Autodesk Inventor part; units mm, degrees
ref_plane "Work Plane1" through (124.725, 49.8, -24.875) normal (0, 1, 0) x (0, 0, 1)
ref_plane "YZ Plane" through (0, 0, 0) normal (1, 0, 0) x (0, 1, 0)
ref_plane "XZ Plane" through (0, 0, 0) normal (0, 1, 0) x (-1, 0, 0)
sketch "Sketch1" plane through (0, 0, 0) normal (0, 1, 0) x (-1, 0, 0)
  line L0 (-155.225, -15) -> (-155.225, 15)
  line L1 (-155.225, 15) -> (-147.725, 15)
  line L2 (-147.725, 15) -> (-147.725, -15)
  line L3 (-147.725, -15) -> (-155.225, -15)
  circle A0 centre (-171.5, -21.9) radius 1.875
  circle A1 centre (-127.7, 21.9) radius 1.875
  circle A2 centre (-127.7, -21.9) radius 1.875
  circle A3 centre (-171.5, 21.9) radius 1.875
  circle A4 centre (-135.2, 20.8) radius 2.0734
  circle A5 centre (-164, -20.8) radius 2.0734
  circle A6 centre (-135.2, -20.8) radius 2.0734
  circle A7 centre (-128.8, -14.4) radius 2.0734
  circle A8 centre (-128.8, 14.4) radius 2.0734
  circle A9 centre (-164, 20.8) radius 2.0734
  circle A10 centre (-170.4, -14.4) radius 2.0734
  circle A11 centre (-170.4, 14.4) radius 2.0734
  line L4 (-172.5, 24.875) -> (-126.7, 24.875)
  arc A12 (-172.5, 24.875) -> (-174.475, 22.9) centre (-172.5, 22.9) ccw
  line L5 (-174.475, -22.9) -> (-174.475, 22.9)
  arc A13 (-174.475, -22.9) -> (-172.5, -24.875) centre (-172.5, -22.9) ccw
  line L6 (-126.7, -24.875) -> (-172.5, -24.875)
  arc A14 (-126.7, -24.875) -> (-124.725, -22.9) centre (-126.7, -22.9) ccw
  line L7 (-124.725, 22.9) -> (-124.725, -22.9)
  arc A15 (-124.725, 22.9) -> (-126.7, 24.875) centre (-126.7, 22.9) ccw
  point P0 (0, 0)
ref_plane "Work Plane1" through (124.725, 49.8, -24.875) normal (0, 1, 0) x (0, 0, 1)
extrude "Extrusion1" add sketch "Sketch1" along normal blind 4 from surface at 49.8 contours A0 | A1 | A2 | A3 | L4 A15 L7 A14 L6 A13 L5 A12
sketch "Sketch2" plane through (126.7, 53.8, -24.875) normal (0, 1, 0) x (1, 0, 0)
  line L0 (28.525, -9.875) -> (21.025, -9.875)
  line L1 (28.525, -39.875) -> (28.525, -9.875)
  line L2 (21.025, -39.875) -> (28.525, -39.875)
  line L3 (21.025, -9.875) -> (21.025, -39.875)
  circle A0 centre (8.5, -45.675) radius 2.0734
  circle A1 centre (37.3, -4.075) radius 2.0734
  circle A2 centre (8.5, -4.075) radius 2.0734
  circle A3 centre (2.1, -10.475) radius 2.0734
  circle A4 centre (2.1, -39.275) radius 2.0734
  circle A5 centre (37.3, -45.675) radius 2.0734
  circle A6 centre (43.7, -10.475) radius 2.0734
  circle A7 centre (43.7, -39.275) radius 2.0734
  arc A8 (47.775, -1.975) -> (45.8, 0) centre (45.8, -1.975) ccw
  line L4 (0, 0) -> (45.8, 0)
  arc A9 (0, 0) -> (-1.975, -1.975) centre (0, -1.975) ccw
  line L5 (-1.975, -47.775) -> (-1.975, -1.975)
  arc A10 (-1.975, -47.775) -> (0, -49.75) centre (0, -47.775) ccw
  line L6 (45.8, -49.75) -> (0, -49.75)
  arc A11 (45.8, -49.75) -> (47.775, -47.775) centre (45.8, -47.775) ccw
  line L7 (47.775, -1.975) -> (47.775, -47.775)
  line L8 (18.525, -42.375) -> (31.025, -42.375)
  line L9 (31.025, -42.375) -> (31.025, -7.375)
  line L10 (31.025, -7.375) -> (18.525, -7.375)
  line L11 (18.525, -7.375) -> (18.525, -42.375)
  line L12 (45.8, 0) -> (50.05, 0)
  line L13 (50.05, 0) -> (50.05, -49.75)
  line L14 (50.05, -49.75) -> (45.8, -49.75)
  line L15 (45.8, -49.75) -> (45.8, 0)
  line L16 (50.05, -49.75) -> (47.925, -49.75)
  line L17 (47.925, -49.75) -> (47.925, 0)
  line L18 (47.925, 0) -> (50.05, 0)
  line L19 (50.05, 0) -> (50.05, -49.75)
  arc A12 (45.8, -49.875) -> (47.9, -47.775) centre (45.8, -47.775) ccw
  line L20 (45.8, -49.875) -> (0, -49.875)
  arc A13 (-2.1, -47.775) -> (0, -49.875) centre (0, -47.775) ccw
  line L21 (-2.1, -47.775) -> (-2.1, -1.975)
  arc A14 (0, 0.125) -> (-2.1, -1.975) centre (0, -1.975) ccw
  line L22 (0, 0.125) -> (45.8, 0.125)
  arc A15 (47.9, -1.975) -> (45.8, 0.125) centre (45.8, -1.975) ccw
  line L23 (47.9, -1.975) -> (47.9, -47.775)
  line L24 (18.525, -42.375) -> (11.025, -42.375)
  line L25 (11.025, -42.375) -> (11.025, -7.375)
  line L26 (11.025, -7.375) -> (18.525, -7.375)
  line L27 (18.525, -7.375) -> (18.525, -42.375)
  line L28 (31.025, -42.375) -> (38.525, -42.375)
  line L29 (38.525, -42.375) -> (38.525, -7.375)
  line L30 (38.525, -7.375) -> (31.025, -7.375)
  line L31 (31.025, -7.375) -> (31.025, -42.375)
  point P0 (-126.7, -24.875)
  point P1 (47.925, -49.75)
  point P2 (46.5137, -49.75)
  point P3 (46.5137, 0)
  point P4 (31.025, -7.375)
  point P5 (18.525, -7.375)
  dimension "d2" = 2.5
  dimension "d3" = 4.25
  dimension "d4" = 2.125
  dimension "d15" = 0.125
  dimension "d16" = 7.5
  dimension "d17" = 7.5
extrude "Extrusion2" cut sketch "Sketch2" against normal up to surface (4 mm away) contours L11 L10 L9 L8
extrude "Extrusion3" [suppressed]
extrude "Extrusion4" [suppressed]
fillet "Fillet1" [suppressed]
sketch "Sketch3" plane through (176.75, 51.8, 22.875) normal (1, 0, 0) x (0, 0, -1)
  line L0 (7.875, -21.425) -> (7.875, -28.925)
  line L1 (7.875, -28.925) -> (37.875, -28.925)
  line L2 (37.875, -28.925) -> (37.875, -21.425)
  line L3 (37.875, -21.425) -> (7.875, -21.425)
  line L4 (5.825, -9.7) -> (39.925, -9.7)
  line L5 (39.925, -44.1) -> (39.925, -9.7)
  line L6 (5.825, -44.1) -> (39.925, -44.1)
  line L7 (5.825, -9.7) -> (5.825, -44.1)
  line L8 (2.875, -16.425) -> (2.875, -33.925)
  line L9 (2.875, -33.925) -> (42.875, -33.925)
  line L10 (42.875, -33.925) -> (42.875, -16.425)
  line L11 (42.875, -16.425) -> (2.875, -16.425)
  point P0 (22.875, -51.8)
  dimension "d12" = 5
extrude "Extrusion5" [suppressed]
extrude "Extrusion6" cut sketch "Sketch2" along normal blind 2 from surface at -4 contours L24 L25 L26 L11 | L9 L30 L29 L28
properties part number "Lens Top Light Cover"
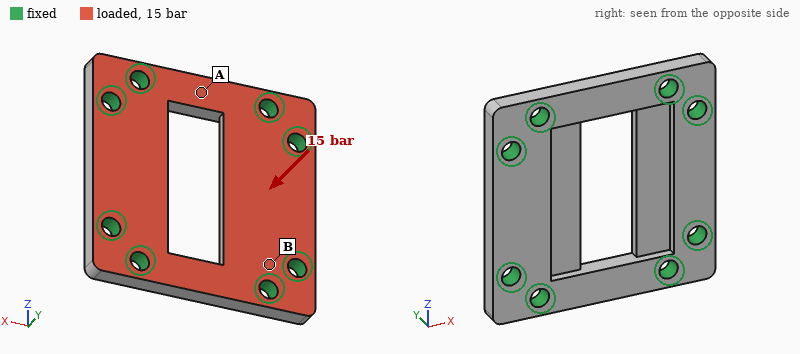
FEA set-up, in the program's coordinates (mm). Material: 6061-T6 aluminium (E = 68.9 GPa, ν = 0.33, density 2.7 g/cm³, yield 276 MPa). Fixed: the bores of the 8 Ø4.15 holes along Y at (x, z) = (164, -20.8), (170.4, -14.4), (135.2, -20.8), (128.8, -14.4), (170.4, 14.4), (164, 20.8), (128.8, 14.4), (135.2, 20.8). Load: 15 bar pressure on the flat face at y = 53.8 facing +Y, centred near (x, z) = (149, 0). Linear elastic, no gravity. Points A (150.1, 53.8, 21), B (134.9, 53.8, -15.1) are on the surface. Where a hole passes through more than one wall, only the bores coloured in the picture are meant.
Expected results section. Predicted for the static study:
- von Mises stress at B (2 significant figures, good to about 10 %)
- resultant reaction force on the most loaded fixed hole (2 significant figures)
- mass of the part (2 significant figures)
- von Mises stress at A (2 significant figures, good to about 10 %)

37 MPa
410 N
18 g
17 MPa
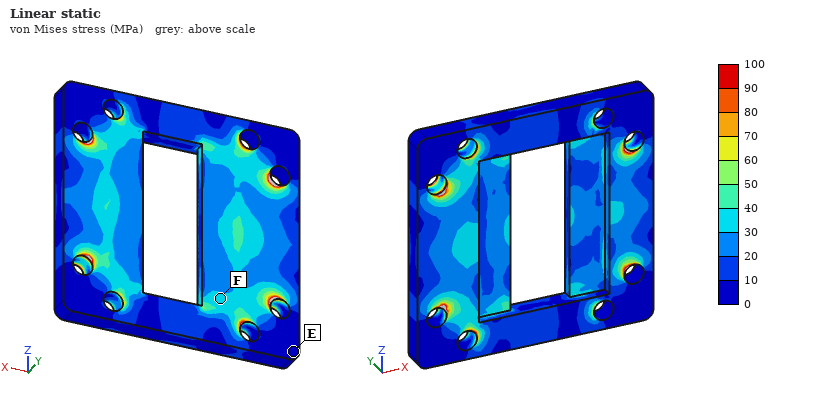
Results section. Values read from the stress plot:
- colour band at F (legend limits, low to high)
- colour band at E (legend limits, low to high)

30 to 40 MPa
0 to 10 MPa
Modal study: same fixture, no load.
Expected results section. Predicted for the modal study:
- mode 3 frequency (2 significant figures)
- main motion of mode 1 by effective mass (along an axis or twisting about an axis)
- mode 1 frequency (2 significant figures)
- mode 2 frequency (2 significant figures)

26 kHz
along Y
15 kHz
17 kHz
